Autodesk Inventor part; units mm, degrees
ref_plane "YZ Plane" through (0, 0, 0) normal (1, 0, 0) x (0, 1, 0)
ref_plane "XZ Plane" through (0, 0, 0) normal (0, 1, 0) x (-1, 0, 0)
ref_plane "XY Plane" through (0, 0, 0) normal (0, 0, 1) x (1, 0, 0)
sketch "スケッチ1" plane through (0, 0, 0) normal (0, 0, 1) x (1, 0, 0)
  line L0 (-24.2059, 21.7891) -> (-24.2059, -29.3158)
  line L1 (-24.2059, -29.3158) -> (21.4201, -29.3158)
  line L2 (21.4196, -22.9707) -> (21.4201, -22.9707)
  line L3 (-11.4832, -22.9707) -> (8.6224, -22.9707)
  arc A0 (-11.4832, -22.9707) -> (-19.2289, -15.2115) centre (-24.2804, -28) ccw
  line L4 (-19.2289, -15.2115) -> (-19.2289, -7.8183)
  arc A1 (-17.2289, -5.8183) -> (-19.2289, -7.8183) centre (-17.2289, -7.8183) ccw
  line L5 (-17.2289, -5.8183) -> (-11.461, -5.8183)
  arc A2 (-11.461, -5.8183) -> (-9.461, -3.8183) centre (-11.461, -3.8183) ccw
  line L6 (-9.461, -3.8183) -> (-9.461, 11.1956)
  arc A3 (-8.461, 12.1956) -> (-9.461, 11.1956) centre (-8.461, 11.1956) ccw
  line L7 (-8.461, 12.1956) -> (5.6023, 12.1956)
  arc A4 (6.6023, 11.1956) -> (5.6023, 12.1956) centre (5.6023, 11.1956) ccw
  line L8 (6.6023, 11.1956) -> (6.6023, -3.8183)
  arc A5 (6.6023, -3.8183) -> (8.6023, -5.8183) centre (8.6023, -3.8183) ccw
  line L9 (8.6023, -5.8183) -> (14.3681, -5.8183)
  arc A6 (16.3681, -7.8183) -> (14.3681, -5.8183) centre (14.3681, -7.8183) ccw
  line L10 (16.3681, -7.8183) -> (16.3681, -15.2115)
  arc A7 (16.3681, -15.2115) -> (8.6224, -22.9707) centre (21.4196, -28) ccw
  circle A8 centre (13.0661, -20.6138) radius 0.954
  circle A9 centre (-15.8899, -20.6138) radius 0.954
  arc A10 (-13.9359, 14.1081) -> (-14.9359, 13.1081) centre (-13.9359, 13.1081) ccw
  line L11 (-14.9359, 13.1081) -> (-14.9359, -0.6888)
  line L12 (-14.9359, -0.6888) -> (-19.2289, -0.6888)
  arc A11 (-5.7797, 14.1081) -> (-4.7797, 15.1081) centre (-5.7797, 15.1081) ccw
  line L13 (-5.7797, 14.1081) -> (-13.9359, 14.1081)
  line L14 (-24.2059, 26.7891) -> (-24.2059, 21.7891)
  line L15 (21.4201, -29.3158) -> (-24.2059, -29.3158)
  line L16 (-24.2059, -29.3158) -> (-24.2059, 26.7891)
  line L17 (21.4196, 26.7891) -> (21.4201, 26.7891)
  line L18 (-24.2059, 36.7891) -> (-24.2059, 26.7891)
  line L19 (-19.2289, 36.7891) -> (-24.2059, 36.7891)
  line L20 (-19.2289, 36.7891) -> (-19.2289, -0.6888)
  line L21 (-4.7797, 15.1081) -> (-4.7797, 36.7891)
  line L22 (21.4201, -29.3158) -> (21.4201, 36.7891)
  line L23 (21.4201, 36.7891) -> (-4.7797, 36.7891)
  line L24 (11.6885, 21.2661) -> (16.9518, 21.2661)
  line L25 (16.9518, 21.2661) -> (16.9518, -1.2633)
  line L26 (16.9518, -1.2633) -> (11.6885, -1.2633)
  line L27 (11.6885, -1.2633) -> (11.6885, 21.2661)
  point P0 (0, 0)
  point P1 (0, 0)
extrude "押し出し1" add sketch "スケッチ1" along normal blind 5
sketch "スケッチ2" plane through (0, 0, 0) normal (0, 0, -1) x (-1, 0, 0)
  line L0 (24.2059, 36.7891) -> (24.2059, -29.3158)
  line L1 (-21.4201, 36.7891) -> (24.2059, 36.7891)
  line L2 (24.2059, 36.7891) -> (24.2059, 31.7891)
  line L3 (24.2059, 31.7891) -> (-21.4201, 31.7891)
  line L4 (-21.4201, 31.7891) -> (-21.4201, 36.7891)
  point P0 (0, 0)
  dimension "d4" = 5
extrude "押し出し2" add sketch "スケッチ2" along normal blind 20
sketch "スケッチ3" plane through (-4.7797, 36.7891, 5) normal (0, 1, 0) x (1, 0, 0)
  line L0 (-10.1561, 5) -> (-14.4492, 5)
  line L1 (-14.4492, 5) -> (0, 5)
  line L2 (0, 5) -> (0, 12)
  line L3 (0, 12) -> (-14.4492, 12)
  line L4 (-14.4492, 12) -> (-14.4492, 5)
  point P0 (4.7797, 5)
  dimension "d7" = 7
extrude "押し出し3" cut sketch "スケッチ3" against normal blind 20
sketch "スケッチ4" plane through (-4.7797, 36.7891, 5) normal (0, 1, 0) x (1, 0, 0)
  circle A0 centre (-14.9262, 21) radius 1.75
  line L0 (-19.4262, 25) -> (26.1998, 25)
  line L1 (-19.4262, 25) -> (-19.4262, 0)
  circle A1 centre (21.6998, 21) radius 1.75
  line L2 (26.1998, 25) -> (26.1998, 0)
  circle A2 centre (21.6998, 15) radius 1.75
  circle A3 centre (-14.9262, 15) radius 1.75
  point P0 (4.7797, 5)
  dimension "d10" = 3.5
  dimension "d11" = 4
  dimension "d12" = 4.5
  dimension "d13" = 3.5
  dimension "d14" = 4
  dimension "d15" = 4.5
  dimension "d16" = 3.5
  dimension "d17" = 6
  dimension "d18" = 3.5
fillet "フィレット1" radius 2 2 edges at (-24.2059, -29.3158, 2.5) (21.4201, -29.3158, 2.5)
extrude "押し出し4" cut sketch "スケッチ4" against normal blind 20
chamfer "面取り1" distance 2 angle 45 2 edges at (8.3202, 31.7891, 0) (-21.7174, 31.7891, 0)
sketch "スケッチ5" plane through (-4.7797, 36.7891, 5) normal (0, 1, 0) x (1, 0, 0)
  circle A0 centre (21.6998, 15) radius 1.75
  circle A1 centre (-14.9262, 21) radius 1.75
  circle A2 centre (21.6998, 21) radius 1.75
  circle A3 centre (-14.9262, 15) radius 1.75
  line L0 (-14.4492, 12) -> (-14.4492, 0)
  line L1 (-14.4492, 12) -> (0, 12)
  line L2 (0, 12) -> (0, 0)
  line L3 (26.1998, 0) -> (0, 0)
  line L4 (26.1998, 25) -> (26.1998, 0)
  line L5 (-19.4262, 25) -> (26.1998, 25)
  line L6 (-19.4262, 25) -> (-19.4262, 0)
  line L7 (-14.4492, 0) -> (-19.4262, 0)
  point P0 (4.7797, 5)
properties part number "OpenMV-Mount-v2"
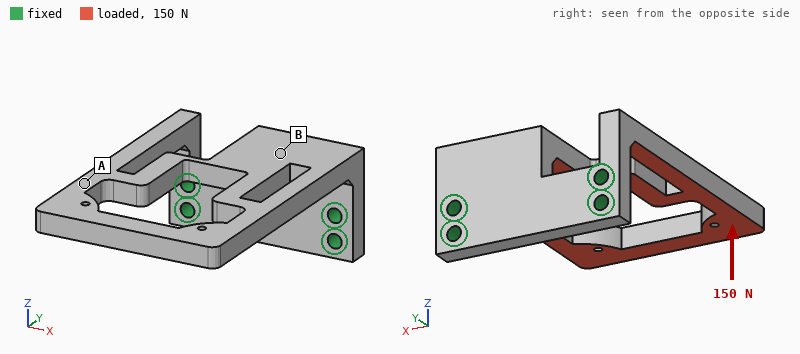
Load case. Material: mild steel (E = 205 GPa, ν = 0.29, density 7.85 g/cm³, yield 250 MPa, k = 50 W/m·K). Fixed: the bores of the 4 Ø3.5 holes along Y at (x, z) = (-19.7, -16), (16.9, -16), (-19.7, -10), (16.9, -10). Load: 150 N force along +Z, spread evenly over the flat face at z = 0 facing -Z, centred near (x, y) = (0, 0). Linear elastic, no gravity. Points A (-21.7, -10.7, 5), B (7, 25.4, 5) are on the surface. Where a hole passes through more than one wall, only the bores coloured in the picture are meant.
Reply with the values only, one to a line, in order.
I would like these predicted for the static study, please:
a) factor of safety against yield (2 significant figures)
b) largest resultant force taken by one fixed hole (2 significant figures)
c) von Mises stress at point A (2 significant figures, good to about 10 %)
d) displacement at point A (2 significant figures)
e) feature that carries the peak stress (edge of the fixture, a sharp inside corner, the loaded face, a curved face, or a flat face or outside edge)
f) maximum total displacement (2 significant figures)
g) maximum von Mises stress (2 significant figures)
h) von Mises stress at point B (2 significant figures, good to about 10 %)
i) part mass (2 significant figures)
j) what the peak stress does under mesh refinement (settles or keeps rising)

2.0
170 N
8.6 MPa
0.11 mm
the loaded face
0.18 mm
120 MPa
25 MPa
97 g
settles
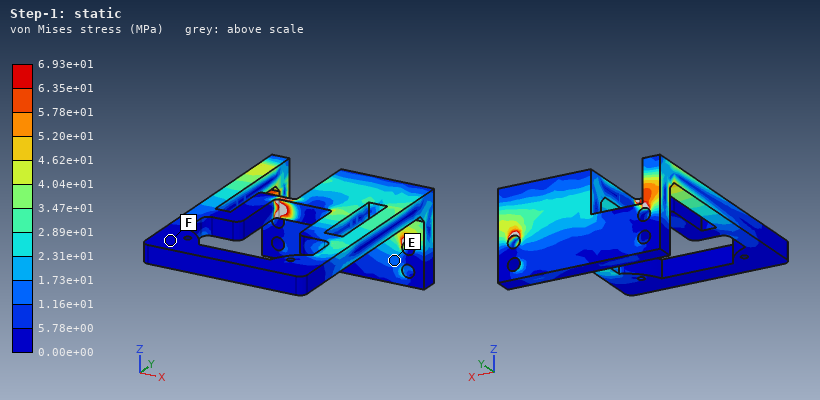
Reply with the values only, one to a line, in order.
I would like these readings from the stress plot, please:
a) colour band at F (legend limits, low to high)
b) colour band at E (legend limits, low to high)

0.00e+00 to 5.78e+00 MPa
1.16e+01 to 1.73e+01 MPa
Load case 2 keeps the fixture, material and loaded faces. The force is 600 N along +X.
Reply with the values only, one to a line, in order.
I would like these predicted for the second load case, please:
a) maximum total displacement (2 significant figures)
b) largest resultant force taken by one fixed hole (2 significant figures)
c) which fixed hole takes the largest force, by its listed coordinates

94 µm
760 N
(16.9, -10)
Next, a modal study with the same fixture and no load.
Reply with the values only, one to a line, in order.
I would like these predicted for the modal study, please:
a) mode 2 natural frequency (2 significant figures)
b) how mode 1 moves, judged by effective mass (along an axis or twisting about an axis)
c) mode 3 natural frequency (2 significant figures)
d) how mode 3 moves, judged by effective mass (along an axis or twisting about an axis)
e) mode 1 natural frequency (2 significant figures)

1800 Hz
along Z
2500 Hz
along X
750 Hz
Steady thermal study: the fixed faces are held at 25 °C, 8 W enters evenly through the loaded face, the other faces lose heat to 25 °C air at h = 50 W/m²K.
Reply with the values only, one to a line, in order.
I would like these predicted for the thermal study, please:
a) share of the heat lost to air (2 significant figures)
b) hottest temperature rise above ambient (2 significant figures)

53 %
30 K
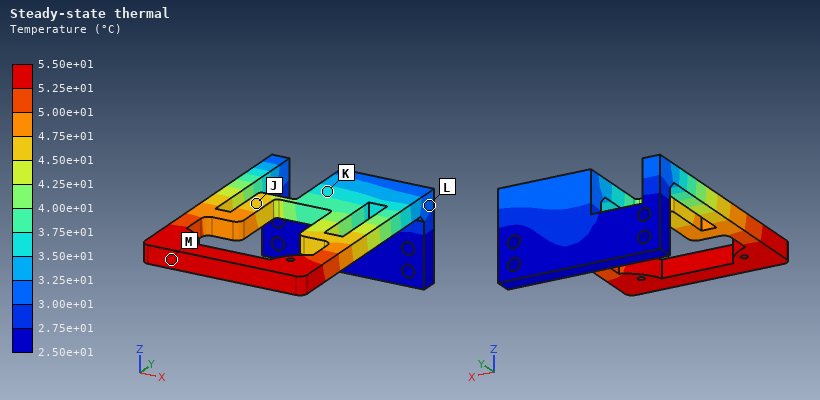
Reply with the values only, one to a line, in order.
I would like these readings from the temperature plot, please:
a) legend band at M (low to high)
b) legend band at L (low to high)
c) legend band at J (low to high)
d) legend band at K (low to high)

5.25e+01 to 5.50e+01 °C
3.00e+01 to 3.25e+01 °C
4.50e+01 to 4.75e+01 °C
3.50e+01 to 3.75e+01 °C
